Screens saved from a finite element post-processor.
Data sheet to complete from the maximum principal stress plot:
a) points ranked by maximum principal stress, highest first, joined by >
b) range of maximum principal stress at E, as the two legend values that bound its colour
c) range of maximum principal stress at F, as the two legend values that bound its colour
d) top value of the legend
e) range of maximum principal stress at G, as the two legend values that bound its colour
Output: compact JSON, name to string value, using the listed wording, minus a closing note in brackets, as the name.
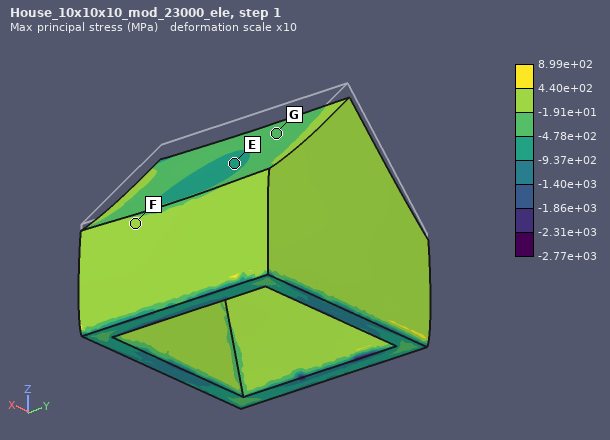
{"points ranked by maximum principal stress, highest first, joined by >": "F > G > E", "range of maximum principal stress at E, as the two legend values that bound its colour": "-9.37e+02 to -4.78e+02 MPa", "range of maximum principal stress at F, as the two legend values that bound its colour": "-1.91e+01 to 4.40e+02 MPa", "top value of the legend": "8.99e+02 MPa", "range of maximum principal stress at G, as the two legend values that bound its colour": "-4.78e+02 to -1.91e+01 MPa"}
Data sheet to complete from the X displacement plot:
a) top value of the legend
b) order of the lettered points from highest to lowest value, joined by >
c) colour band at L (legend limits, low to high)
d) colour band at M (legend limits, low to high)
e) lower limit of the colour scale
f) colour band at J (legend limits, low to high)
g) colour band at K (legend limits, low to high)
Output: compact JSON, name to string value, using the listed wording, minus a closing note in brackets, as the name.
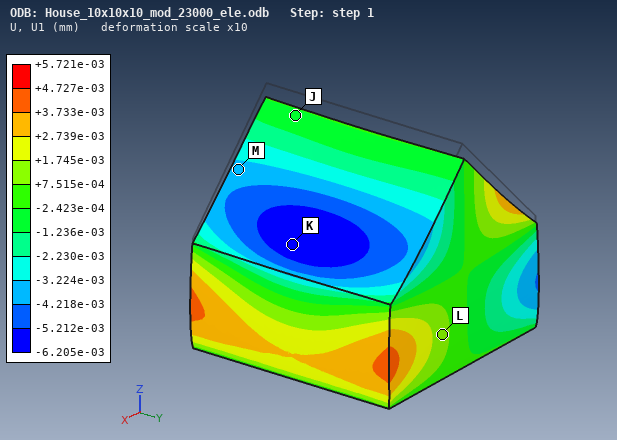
{"top value of the legend": "+5.721e-03 mm", "order of the lettered points from highest to lowest value, joined by >": "L > J > M > K", "colour band at L": "+7.515e-04 to +1.745e-03 mm", "colour band at M": "-4.218e-03 to -3.224e-03 mm", "lower limit of the colour scale": "-6.205e-03 mm", "colour band at J": "-1.236e-03 to -2.423e-04 mm", "colour band at K": "-6.205e-03 to -5.212e-03 mm"}
